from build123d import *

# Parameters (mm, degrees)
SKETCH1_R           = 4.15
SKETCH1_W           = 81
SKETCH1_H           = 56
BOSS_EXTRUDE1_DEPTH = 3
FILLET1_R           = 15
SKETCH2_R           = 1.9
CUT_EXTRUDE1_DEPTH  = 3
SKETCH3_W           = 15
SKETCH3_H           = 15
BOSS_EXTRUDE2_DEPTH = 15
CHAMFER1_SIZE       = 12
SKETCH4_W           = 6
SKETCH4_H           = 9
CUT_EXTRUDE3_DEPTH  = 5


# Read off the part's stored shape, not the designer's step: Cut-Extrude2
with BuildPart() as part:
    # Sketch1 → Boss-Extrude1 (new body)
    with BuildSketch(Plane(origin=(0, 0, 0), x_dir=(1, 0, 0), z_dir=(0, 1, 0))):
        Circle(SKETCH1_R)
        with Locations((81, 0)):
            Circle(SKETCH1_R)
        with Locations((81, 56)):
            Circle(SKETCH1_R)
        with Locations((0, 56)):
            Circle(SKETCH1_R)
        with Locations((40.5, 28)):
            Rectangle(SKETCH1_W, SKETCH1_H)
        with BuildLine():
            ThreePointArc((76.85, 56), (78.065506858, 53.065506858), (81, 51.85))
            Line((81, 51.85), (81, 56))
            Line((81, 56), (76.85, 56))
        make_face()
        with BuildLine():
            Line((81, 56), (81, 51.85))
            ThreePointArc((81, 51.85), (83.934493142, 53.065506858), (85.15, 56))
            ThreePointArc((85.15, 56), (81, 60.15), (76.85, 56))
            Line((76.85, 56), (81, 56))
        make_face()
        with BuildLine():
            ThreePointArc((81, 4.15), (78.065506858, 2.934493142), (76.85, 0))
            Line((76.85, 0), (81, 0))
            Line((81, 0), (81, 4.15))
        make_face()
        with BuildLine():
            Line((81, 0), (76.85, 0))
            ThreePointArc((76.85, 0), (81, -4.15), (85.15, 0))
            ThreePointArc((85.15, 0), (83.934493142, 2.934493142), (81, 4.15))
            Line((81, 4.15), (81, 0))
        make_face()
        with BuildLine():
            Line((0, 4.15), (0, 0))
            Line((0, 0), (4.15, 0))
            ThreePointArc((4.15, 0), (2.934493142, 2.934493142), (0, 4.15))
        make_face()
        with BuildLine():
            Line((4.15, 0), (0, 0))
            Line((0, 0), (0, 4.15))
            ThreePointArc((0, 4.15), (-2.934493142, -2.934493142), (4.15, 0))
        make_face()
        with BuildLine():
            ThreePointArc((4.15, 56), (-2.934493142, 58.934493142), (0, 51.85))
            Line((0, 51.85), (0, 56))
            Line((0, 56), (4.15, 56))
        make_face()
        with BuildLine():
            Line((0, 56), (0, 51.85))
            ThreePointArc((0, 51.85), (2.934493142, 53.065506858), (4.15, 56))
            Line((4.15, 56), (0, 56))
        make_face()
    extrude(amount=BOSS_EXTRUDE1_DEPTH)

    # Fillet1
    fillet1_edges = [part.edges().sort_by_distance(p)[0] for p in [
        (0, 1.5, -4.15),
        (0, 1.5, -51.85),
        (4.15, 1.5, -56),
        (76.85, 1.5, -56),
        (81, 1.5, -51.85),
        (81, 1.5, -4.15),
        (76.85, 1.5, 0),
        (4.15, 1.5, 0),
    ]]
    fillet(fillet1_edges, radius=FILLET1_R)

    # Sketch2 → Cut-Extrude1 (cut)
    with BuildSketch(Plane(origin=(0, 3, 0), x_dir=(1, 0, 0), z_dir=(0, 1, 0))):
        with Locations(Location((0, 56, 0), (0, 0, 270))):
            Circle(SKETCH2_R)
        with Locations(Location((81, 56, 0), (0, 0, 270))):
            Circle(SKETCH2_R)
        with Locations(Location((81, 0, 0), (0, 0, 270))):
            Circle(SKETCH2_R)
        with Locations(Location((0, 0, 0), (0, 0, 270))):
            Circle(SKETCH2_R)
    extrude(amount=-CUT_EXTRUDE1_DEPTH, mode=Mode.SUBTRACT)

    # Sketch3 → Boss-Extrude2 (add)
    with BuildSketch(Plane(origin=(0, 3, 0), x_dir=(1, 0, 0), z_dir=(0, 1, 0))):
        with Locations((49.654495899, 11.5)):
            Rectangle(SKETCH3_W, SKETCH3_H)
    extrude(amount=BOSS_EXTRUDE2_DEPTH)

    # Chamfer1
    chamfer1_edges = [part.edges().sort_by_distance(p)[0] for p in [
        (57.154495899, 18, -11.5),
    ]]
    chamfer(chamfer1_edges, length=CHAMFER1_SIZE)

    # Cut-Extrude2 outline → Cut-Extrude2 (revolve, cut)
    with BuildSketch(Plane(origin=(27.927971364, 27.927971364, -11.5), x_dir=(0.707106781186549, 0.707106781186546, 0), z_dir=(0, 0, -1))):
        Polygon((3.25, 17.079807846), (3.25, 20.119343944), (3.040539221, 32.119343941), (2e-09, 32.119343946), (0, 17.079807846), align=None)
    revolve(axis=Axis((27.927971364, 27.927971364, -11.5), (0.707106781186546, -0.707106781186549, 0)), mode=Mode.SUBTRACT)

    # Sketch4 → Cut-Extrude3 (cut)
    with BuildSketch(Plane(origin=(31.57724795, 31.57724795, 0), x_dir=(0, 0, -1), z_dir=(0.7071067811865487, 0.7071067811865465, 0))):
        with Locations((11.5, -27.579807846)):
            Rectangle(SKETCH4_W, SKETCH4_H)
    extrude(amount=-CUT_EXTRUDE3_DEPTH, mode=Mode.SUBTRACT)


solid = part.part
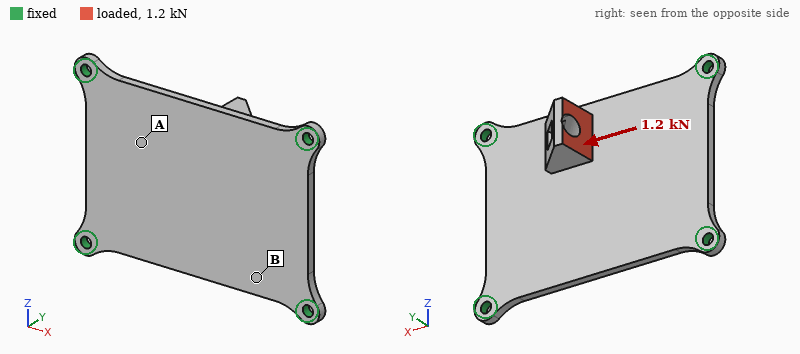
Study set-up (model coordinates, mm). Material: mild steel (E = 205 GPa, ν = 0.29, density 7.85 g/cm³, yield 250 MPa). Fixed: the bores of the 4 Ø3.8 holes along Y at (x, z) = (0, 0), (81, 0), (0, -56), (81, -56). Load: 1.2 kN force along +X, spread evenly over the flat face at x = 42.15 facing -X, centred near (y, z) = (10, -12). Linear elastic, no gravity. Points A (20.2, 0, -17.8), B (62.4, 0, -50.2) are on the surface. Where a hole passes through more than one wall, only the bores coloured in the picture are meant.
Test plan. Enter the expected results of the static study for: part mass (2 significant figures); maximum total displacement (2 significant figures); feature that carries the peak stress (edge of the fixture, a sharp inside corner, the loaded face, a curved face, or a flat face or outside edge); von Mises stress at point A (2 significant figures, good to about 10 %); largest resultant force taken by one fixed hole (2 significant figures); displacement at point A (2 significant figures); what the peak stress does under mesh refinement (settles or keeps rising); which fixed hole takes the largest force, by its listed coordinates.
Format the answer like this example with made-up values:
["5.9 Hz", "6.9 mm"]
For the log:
["120 g", "60 µm", "edge of the fixture", "20 MPa", "470 N", "29 µm", "keeps rising", "(81, 0)"]
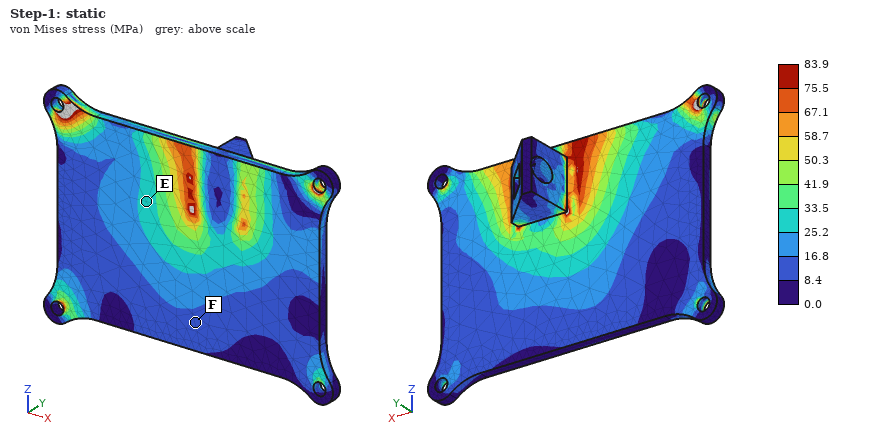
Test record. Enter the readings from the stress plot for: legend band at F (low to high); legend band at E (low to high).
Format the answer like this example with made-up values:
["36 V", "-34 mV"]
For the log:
["8.4 to 16.8 MPa", "25.2 to 33.5 MPa"]
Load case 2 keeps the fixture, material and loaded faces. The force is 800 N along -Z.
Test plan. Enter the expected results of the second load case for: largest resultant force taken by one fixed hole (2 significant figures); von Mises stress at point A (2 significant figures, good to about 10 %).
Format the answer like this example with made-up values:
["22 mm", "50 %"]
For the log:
["310 N", "19 MPa"]
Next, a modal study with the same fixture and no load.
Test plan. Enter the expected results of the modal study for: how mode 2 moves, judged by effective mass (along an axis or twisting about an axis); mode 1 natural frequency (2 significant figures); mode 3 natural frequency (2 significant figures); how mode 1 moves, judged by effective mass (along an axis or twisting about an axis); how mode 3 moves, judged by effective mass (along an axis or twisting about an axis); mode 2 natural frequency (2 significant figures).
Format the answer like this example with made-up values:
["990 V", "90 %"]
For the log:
["twisting about X", "1700 Hz", "4300 Hz", "along Y", "twisting about Z", "3000 Hz"]
